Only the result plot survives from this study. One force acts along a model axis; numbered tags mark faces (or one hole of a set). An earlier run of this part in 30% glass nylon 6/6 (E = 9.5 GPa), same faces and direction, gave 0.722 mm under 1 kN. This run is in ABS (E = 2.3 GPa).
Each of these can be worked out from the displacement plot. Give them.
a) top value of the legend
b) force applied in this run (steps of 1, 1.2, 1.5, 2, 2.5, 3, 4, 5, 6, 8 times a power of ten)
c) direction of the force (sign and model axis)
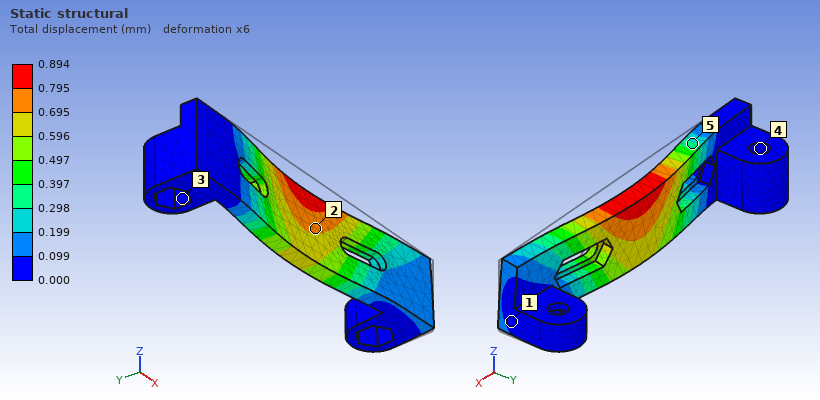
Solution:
0.894 mm
300 N
+Y
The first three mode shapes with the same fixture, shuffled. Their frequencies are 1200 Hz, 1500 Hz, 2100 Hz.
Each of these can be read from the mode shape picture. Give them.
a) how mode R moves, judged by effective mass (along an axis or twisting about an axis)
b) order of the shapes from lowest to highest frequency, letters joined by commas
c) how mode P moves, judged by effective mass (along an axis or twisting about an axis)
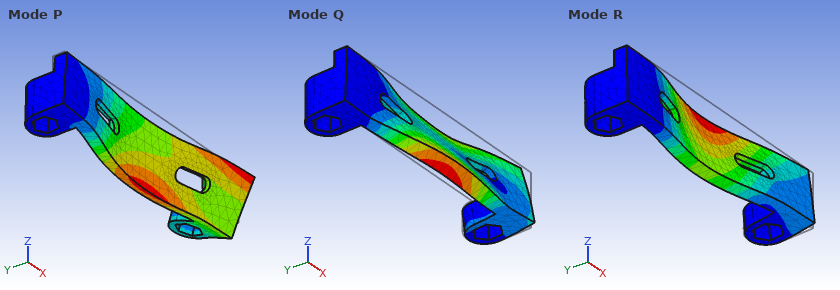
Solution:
along Y
R, P, Q
along Z
